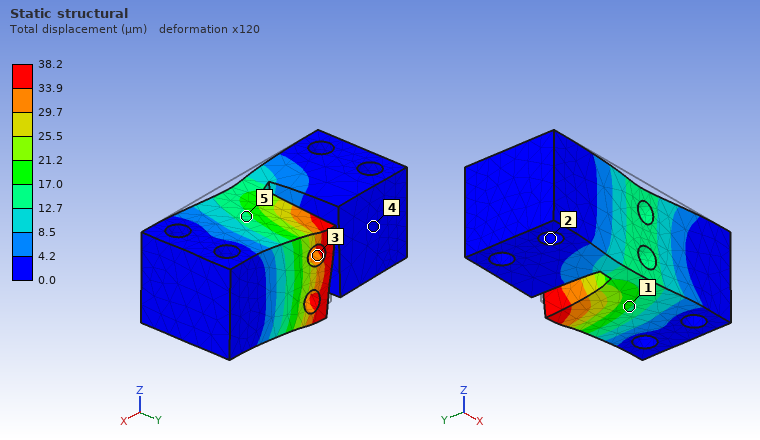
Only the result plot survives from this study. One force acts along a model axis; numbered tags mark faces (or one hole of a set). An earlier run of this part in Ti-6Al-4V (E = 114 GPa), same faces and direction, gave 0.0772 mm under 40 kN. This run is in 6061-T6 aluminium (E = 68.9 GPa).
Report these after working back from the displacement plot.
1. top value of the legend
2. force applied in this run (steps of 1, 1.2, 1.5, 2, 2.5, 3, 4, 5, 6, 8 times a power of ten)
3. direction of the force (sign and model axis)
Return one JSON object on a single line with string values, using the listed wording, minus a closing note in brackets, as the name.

{"top value of the legend": "38.2 µm", "force applied in this run": "12 kN", "direction of the force": "-Z"}
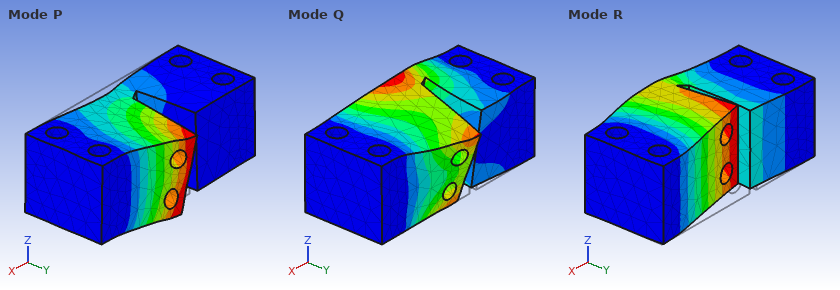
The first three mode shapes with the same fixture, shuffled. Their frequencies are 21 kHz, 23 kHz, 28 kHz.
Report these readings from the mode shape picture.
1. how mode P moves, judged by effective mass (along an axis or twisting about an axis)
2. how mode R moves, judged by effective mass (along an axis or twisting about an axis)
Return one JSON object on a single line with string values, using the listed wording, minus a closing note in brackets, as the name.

{"how mode P moves, judged by effective mass": "along Z", "how mode R moves, judged by effective mass": "along Y"}
